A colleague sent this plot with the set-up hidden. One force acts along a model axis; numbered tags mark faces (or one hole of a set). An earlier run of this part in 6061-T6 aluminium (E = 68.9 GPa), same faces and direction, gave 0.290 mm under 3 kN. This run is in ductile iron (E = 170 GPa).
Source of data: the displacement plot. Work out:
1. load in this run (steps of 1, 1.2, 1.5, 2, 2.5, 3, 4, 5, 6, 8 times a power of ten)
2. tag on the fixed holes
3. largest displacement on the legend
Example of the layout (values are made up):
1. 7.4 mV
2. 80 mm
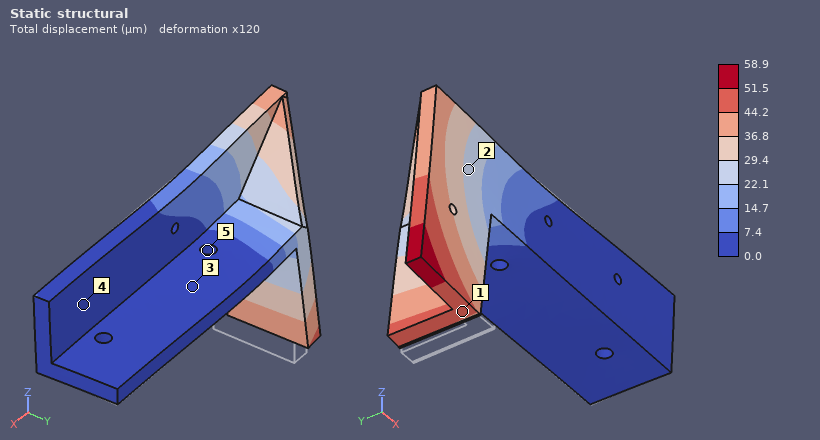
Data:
1. 1.5 kN
2. 5
3. 58.9 µm
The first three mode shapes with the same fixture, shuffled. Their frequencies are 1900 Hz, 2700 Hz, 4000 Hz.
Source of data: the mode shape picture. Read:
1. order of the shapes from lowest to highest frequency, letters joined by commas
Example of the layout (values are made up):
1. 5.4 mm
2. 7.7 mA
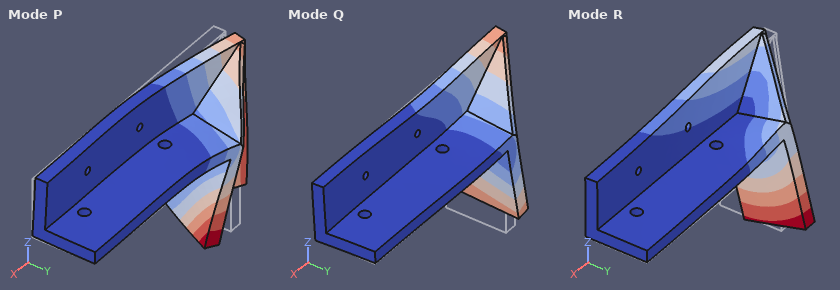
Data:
1. R, Q, P
